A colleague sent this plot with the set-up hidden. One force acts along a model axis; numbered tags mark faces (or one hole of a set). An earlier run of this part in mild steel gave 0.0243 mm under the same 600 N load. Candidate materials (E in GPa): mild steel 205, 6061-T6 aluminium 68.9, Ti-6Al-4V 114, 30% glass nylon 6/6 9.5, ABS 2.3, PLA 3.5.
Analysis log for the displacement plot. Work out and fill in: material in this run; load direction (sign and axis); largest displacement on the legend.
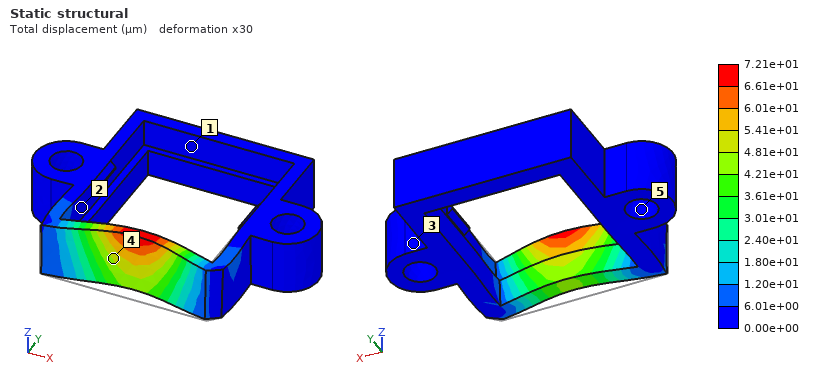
6061-T6 aluminium
+Y
7.21e+01 µm
